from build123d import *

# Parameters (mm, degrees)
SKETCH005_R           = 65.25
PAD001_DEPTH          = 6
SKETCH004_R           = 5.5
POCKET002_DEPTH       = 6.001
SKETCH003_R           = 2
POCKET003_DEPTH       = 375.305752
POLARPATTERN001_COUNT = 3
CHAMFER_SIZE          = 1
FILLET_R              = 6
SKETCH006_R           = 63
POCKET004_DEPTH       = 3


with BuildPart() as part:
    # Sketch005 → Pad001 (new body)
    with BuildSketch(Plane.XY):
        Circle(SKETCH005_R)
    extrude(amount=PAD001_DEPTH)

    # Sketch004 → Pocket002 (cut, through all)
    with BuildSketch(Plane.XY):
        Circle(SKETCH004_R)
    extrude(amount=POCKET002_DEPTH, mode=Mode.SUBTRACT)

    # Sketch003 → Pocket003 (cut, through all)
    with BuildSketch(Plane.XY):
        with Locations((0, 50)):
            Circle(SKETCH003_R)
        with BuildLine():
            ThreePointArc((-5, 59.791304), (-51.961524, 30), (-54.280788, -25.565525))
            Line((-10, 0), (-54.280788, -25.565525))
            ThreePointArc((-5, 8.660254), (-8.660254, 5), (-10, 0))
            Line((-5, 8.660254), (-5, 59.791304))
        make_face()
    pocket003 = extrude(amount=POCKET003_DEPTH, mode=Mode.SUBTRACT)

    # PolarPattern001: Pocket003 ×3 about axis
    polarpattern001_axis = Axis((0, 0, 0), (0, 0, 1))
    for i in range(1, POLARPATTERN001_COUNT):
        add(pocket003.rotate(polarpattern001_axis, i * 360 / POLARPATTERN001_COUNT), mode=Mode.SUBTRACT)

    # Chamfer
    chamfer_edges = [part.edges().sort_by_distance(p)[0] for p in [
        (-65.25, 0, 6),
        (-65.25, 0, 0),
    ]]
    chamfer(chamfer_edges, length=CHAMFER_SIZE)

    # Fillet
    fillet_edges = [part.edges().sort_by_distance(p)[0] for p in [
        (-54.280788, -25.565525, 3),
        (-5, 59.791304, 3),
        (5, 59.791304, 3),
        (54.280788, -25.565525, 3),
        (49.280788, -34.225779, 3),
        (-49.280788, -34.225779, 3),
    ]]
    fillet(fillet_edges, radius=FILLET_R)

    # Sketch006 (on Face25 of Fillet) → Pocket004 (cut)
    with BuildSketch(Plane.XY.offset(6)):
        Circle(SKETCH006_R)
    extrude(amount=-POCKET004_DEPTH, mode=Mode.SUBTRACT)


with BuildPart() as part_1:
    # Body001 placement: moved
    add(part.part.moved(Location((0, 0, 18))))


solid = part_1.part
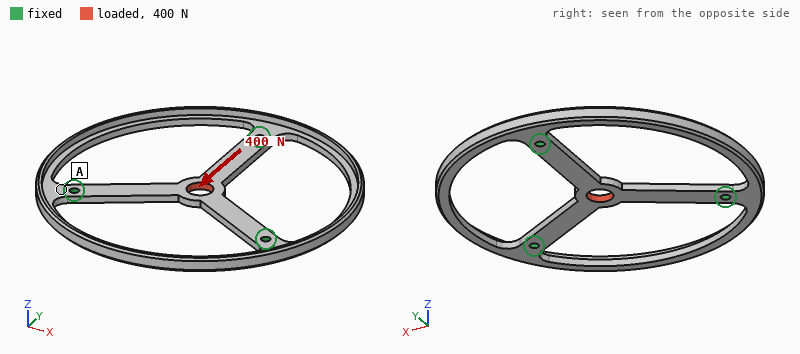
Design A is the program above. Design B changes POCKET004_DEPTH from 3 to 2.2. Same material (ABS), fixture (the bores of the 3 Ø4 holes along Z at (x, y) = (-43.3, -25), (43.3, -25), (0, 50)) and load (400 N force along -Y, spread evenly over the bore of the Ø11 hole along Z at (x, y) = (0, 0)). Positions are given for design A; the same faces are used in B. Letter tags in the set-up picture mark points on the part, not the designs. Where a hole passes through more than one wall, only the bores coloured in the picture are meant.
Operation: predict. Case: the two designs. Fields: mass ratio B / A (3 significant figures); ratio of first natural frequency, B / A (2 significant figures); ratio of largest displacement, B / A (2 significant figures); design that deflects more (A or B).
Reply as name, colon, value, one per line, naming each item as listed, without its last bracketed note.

mass ratio B / A: 1.17
ratio of first natural frequency, B / A: 1.1
ratio of largest displacement, B / A: 0.79
design that deflects more: A
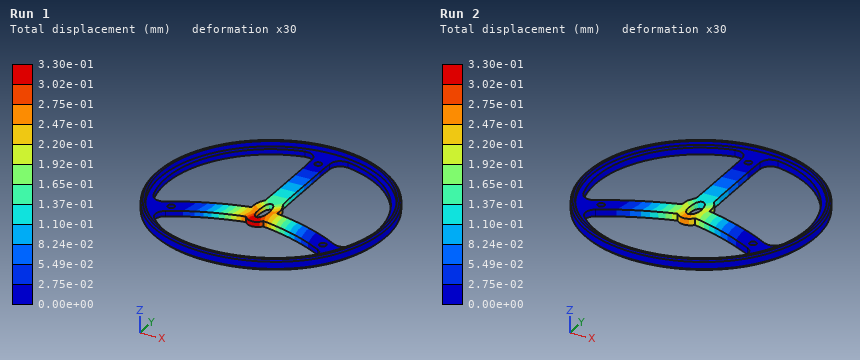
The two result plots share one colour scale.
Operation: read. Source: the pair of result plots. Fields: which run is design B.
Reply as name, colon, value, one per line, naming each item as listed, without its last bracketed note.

which run is design B: Run 2
